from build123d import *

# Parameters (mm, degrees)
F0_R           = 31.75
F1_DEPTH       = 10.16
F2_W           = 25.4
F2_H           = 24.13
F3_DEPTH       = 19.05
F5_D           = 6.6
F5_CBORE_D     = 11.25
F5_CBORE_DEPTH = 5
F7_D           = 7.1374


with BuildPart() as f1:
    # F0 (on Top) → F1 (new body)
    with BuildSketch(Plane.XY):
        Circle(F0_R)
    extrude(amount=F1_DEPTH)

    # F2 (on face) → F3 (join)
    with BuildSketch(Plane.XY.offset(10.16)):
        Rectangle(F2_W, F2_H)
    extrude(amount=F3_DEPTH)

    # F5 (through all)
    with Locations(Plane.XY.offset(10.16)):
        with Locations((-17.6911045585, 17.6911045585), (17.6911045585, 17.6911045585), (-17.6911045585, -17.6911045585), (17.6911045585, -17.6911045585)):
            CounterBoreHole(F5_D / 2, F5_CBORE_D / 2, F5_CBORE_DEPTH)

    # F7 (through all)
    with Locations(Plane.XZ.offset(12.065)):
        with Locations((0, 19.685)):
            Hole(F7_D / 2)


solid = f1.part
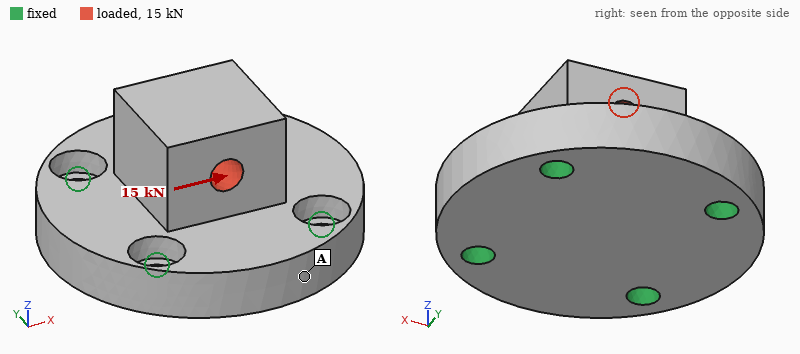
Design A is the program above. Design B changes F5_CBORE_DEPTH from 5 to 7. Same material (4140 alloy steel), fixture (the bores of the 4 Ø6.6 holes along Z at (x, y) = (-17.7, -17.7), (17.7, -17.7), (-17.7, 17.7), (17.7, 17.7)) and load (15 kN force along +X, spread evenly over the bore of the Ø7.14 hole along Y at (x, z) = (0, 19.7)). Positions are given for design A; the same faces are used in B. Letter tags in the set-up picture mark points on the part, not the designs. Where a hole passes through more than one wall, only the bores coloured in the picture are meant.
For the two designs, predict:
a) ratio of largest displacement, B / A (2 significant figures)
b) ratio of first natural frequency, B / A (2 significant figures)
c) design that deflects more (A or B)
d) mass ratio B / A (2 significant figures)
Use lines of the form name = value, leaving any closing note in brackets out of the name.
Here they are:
ratio of largest displacement, B / A = 1.2
ratio of first natural frequency, B / A = 0.86
design that deflects more = B
mass ratio B / A = 0.99
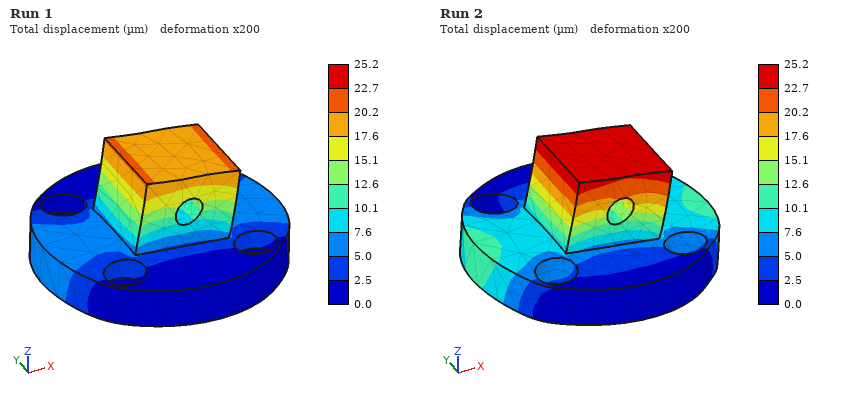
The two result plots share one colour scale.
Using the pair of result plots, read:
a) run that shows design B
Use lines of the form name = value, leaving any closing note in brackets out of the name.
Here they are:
run that shows design B = Run 2
